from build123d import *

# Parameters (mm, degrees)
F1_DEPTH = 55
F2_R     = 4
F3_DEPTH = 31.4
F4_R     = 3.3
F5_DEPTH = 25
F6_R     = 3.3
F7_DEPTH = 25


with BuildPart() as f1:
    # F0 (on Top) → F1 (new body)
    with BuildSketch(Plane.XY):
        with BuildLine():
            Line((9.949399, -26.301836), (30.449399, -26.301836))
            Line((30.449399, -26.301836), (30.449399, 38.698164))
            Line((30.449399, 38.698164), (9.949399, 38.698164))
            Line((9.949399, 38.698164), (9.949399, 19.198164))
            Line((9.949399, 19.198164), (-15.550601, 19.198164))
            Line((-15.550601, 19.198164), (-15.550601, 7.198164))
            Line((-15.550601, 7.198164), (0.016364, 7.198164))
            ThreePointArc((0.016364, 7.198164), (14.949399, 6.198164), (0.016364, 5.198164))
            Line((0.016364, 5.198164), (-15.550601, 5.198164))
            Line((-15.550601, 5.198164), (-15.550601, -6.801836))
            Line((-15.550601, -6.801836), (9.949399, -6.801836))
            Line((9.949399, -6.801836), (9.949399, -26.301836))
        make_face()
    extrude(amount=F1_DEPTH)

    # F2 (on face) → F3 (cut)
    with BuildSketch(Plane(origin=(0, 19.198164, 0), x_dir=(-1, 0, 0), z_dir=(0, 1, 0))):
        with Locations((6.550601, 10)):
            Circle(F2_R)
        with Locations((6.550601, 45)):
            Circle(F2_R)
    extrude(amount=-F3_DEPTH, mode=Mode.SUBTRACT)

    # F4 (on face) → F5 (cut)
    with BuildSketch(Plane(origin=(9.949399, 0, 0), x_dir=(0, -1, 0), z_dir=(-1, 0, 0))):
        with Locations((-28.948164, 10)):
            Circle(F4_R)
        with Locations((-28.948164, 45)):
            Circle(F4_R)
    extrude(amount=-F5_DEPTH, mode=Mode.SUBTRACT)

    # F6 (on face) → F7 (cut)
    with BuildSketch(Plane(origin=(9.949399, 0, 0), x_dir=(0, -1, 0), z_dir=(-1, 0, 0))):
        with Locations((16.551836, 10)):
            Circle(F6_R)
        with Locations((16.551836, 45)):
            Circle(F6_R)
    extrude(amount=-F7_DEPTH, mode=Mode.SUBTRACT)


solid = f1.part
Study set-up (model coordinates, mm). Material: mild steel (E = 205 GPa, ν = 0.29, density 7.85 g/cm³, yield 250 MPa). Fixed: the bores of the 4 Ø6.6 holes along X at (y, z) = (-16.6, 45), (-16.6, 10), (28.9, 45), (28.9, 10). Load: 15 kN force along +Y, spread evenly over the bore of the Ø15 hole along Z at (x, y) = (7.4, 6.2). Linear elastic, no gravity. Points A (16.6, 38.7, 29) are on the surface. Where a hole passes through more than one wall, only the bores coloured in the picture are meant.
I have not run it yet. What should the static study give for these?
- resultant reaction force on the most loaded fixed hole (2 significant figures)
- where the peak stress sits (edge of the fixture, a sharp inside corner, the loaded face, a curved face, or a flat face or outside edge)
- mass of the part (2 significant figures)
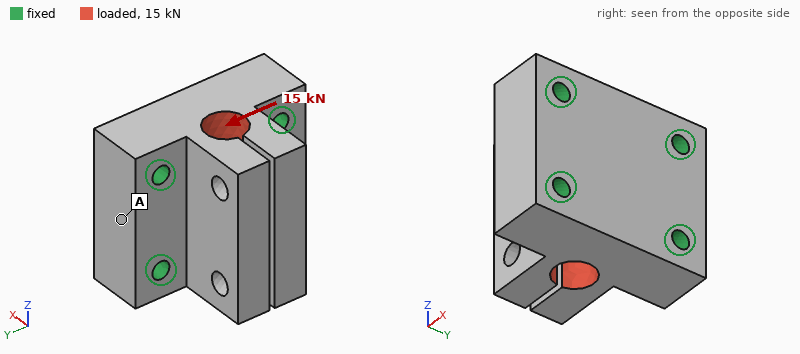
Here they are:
4.2 kN
the loaded face
730 g
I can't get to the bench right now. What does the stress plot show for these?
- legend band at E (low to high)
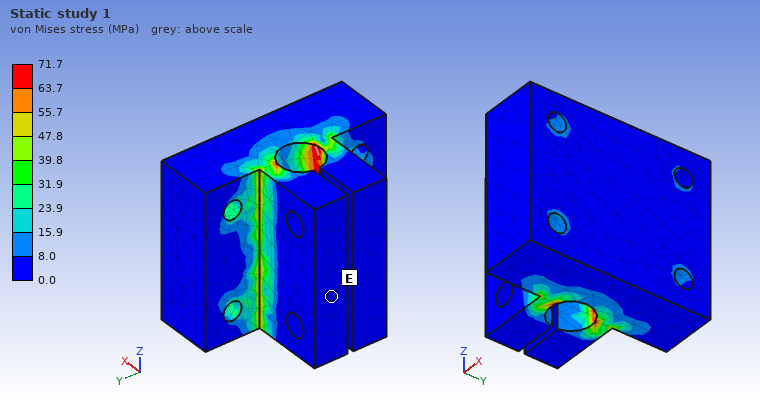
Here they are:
0.0 to 8.0 MPa
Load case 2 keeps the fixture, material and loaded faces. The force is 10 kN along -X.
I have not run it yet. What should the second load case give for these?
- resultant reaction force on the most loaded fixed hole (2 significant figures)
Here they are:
2.5 kN
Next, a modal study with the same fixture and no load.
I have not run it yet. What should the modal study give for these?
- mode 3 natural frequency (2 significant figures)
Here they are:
9500 Hz
